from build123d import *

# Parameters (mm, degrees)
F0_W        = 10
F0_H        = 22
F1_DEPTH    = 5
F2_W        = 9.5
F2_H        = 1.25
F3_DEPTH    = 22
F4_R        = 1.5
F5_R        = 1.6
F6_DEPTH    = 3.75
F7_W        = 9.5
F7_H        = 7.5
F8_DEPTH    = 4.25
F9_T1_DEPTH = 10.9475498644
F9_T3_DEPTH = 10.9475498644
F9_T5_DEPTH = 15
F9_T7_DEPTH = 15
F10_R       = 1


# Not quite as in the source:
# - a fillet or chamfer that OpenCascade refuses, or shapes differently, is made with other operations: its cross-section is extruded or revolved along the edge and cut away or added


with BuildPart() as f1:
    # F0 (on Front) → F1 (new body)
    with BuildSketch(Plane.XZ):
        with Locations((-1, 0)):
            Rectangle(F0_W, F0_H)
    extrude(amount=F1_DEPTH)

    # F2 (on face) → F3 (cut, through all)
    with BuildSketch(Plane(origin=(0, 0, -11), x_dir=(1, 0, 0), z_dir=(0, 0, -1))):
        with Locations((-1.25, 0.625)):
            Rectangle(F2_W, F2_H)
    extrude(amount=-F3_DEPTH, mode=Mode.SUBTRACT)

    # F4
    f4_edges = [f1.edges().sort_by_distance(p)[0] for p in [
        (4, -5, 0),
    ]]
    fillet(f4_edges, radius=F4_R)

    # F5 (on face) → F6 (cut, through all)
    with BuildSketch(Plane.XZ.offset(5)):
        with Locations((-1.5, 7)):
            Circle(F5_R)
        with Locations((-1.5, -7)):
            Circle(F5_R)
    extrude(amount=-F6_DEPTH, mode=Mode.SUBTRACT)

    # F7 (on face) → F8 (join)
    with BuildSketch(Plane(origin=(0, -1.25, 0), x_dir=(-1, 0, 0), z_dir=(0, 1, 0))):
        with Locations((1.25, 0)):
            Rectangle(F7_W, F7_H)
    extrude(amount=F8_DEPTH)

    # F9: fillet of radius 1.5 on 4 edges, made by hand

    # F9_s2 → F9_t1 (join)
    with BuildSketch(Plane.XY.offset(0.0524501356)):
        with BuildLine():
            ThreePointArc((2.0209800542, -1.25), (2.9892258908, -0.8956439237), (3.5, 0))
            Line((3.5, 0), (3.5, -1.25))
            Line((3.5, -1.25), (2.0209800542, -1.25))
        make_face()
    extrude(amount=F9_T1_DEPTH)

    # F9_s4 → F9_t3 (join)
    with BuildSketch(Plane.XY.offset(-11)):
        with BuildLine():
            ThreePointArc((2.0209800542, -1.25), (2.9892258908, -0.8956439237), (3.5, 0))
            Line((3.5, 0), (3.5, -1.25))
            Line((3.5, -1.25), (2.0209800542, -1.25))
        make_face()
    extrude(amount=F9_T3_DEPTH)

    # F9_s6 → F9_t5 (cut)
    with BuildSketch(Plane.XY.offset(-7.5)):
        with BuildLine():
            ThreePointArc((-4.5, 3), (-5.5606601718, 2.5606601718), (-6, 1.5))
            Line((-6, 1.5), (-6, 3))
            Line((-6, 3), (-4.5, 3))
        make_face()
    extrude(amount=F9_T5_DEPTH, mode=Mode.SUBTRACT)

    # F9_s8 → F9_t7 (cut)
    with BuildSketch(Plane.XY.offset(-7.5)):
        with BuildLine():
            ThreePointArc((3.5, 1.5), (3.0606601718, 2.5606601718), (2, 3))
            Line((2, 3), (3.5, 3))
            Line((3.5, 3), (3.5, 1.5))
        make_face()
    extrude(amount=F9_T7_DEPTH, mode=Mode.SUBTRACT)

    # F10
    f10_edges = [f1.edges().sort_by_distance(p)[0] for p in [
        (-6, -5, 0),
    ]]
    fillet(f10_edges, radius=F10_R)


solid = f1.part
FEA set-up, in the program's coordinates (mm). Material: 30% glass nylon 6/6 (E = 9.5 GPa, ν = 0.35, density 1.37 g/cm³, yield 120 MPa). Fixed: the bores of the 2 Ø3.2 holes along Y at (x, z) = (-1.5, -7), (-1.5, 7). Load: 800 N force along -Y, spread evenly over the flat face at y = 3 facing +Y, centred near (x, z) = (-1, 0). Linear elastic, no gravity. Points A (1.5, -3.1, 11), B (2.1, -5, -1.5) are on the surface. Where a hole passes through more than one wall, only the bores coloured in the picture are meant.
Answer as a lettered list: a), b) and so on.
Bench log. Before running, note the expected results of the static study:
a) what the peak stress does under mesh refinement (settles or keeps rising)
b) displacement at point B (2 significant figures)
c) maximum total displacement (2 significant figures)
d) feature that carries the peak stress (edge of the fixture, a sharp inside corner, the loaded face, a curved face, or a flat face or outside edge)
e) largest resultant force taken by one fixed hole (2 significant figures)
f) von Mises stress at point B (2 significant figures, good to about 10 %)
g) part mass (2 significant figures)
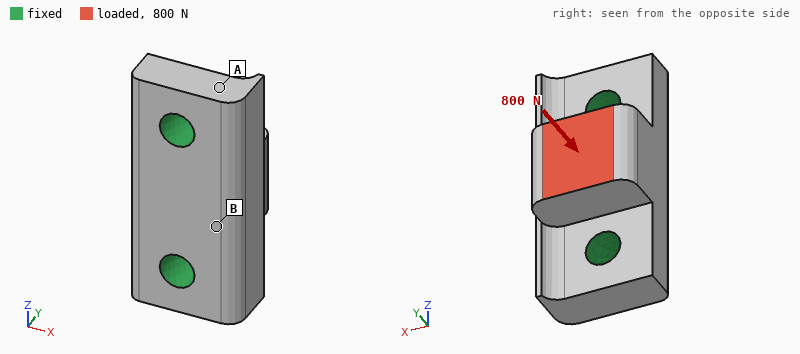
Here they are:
a) keeps rising
b) 21 µm
c) 27 µm
d) edge of the fixture
e) 420 N
f) 15 MPa
g) 1.5 g
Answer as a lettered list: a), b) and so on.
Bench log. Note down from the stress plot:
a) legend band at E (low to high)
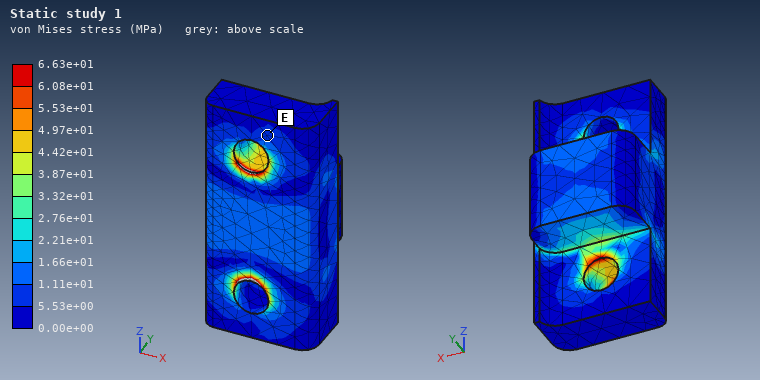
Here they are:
a) 5.53e+00 to 1.11e+01 MPa
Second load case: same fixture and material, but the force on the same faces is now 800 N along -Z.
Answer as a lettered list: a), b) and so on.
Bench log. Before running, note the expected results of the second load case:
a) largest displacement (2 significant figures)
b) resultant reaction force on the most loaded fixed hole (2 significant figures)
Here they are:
a) 65 µm
b) 590 N
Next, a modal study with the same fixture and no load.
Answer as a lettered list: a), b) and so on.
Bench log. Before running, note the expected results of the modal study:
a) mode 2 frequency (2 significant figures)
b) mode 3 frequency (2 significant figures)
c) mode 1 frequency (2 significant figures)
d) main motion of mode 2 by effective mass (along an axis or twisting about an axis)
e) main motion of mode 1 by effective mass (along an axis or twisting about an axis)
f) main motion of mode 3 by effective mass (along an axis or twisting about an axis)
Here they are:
a) 34 kHz
b) 42 kHz
c) 22 kHz
d) along Y
e) along X
f) along Z
